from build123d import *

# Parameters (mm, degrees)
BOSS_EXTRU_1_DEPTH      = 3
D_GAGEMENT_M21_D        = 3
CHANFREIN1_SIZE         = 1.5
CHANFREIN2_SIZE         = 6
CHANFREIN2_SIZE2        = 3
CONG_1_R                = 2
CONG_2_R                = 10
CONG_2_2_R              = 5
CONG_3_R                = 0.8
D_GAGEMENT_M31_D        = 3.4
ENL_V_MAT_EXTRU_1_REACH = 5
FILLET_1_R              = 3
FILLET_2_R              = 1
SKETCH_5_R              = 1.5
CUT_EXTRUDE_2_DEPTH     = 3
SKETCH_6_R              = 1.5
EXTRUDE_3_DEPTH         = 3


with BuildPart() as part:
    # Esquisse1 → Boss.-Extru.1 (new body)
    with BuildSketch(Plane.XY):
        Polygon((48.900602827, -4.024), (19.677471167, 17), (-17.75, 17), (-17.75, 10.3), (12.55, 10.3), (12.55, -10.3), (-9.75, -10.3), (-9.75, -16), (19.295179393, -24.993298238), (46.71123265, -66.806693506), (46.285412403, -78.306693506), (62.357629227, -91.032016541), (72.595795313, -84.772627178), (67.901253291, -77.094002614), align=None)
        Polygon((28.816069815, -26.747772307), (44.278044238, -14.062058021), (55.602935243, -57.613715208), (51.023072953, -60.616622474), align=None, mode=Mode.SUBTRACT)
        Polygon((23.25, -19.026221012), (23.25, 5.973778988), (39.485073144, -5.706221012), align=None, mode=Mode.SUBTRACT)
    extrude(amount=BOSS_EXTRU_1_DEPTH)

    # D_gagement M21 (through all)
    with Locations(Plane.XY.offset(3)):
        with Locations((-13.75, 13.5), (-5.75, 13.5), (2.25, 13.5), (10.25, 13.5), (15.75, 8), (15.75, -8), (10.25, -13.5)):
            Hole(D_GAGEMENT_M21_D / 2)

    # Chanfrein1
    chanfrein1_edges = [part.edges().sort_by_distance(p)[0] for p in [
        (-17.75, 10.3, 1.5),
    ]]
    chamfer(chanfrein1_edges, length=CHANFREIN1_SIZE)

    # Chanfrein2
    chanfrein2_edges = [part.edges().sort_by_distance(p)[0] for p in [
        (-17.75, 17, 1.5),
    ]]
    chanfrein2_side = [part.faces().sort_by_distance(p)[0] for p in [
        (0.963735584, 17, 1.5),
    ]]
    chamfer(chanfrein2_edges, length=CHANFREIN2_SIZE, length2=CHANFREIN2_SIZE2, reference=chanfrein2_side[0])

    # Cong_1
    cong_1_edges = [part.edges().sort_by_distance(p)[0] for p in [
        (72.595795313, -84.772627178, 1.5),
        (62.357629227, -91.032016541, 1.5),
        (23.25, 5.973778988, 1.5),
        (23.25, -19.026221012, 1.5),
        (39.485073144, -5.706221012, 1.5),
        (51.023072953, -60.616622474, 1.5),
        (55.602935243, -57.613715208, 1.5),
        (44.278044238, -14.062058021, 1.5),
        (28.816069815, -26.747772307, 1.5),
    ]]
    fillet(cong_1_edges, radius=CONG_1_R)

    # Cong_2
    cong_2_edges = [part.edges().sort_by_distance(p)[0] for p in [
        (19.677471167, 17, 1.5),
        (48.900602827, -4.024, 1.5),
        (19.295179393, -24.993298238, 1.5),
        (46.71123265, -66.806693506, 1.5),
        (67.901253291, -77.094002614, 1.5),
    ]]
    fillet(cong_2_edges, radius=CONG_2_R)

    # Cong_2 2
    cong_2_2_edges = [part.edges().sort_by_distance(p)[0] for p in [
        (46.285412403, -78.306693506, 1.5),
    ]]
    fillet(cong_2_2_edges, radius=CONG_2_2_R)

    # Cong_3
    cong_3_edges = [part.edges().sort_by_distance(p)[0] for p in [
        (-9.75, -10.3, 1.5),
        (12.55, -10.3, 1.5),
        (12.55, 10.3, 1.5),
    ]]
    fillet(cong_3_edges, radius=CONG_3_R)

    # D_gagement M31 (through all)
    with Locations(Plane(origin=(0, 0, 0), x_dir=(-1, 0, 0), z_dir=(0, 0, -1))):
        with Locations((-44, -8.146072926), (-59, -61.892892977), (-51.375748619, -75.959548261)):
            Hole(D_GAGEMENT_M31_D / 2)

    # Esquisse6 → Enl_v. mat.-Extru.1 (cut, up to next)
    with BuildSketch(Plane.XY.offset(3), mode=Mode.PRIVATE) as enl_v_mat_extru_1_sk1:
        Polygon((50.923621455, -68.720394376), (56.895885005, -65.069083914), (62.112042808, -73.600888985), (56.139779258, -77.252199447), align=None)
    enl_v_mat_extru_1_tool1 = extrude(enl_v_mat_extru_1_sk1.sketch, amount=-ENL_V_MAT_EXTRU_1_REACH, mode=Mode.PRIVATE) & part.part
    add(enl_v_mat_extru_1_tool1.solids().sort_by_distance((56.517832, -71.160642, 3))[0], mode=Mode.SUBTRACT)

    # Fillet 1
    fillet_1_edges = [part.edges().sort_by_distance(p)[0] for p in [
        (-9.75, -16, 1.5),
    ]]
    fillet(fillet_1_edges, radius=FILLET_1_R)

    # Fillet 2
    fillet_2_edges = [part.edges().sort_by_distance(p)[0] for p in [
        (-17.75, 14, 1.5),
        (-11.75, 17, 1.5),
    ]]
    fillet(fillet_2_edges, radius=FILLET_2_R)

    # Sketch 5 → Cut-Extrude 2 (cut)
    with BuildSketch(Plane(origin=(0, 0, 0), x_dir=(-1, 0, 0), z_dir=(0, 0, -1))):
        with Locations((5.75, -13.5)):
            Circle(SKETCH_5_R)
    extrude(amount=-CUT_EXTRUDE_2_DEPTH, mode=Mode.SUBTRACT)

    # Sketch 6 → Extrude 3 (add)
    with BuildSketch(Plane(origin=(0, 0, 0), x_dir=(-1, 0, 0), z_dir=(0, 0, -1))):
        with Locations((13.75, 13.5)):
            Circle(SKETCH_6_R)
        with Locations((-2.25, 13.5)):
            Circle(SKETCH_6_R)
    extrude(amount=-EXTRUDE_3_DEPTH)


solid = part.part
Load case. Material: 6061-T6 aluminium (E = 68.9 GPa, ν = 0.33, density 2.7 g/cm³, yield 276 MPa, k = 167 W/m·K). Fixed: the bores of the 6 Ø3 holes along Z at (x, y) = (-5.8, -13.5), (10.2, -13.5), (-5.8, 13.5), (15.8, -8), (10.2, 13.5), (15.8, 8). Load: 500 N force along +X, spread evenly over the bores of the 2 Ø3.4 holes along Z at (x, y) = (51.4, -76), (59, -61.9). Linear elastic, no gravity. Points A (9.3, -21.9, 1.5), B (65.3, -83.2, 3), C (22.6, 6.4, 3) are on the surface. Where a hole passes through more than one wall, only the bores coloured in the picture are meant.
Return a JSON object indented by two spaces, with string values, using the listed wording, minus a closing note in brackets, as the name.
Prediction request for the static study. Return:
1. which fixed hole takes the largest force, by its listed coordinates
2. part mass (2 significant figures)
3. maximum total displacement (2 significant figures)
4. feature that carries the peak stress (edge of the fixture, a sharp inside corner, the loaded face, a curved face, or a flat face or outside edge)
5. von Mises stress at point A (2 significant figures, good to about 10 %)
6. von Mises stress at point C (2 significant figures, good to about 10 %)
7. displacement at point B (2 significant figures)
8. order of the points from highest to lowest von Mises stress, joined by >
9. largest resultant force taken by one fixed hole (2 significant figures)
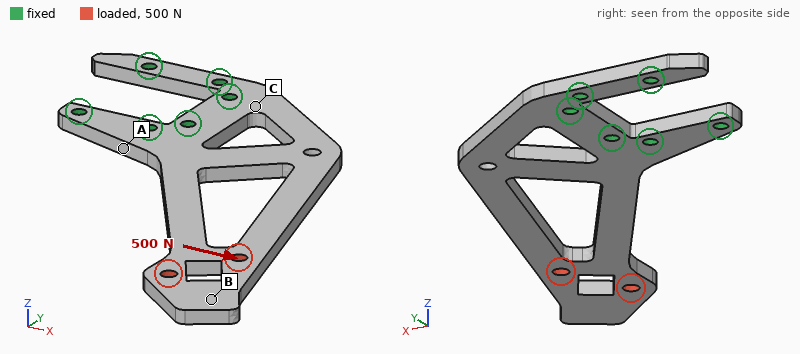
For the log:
{
  "which fixed hole takes the largest force, by its listed coordinates": "(10.2, -13.5)",
  "part mass": "19 g",
  "maximum total displacement": "0.32 mm",
  "feature that carries the peak stress": "a curved face",
  "von Mises stress at point A": "42 MPa",
  "von Mises stress at point C": "31 MPa",
  "displacement at point B": "0.32 mm",
  "order of the points from highest to lowest von Mises stress, joined by >": "A > C > B",
  "largest resultant force taken by one fixed hole": "1.1 kN"
}
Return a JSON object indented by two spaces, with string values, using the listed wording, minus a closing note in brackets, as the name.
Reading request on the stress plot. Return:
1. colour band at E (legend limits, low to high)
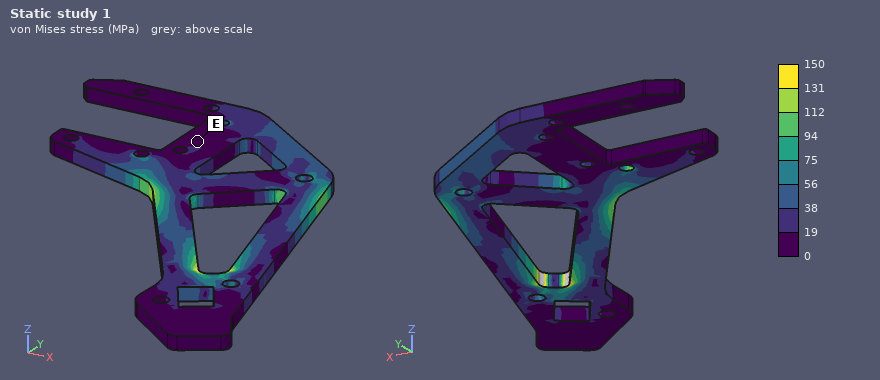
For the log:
{
  "colour band at E": "0 to 19 MPa"
}
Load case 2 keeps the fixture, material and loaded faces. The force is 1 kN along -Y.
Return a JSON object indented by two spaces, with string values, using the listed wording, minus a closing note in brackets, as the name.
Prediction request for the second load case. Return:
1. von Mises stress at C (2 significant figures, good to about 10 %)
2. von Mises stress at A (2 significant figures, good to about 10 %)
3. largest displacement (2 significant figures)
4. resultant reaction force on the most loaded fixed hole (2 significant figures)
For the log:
{
  "von Mises stress at C": "45 MPa",
  "von Mises stress at A": "55 MPa",
  "largest displacement": "0.32 mm",
  "resultant reaction force on the most loaded fixed hole": "1.0 kN"
}
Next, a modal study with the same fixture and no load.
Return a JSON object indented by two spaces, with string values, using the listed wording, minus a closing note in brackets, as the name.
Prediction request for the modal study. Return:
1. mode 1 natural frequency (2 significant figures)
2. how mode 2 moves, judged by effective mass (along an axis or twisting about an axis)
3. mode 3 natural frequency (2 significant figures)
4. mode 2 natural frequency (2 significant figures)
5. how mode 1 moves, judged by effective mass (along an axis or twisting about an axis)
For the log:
{
  "mode 1 natural frequency": "290 Hz",
  "how mode 2 moves, judged by effective mass": "along Z",
  "mode 3 natural frequency": "2200 Hz",
  "mode 2 natural frequency": "1400 Hz",
  "how mode 1 moves, judged by effective mass": "along Z"
}
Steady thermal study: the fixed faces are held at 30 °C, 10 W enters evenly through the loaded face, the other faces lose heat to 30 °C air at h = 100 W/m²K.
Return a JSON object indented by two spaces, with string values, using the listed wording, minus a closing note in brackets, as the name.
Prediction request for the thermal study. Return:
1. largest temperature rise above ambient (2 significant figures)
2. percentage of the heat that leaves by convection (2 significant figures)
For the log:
{
  "largest temperature rise above ambient": "39 K",
  "percentage of the heat that leaves by convection": "78 %"
}
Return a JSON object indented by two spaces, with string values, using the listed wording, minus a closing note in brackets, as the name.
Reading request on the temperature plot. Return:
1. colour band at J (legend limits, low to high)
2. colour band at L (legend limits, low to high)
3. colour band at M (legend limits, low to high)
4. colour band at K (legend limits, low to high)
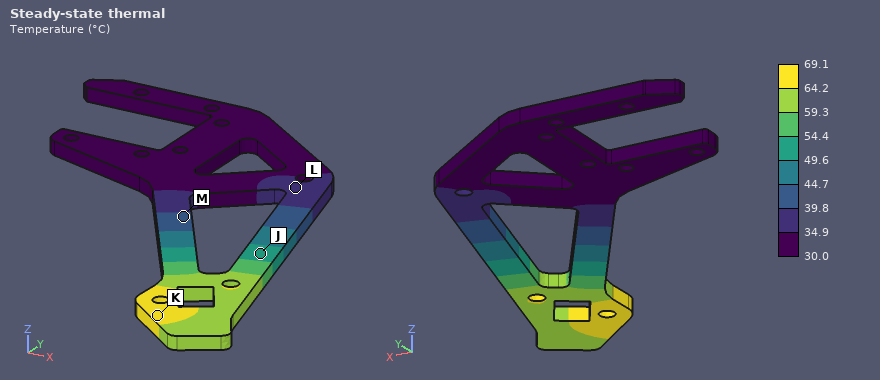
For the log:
{
  "colour band at J": "49.6 to 54.4 °C",
  "colour band at L": "34.9 to 39.8 °C",
  "colour band at M": "39.8 to 44.7 °C",
  "colour band at K": "64.2 to 69.1 °C"
}
